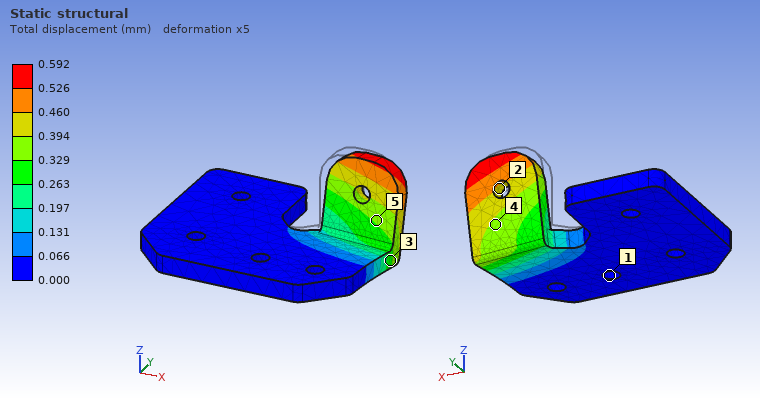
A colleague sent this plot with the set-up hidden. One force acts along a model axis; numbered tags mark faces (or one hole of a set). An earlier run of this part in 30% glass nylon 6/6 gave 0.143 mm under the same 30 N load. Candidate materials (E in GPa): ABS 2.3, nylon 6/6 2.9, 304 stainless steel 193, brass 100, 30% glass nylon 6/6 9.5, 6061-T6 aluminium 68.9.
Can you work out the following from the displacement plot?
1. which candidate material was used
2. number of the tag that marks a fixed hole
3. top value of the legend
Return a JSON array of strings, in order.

["ABS", "1", "0.592 mm"]
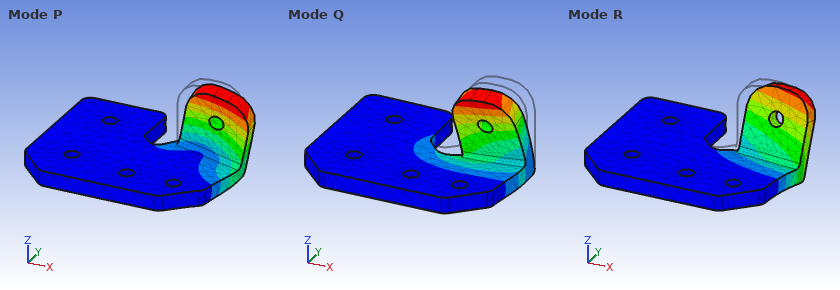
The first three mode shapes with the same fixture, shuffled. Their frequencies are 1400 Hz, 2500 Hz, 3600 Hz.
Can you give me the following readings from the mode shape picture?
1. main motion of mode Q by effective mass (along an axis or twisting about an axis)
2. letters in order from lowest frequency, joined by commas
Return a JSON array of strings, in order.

["along Z", "R, P, Q"]
